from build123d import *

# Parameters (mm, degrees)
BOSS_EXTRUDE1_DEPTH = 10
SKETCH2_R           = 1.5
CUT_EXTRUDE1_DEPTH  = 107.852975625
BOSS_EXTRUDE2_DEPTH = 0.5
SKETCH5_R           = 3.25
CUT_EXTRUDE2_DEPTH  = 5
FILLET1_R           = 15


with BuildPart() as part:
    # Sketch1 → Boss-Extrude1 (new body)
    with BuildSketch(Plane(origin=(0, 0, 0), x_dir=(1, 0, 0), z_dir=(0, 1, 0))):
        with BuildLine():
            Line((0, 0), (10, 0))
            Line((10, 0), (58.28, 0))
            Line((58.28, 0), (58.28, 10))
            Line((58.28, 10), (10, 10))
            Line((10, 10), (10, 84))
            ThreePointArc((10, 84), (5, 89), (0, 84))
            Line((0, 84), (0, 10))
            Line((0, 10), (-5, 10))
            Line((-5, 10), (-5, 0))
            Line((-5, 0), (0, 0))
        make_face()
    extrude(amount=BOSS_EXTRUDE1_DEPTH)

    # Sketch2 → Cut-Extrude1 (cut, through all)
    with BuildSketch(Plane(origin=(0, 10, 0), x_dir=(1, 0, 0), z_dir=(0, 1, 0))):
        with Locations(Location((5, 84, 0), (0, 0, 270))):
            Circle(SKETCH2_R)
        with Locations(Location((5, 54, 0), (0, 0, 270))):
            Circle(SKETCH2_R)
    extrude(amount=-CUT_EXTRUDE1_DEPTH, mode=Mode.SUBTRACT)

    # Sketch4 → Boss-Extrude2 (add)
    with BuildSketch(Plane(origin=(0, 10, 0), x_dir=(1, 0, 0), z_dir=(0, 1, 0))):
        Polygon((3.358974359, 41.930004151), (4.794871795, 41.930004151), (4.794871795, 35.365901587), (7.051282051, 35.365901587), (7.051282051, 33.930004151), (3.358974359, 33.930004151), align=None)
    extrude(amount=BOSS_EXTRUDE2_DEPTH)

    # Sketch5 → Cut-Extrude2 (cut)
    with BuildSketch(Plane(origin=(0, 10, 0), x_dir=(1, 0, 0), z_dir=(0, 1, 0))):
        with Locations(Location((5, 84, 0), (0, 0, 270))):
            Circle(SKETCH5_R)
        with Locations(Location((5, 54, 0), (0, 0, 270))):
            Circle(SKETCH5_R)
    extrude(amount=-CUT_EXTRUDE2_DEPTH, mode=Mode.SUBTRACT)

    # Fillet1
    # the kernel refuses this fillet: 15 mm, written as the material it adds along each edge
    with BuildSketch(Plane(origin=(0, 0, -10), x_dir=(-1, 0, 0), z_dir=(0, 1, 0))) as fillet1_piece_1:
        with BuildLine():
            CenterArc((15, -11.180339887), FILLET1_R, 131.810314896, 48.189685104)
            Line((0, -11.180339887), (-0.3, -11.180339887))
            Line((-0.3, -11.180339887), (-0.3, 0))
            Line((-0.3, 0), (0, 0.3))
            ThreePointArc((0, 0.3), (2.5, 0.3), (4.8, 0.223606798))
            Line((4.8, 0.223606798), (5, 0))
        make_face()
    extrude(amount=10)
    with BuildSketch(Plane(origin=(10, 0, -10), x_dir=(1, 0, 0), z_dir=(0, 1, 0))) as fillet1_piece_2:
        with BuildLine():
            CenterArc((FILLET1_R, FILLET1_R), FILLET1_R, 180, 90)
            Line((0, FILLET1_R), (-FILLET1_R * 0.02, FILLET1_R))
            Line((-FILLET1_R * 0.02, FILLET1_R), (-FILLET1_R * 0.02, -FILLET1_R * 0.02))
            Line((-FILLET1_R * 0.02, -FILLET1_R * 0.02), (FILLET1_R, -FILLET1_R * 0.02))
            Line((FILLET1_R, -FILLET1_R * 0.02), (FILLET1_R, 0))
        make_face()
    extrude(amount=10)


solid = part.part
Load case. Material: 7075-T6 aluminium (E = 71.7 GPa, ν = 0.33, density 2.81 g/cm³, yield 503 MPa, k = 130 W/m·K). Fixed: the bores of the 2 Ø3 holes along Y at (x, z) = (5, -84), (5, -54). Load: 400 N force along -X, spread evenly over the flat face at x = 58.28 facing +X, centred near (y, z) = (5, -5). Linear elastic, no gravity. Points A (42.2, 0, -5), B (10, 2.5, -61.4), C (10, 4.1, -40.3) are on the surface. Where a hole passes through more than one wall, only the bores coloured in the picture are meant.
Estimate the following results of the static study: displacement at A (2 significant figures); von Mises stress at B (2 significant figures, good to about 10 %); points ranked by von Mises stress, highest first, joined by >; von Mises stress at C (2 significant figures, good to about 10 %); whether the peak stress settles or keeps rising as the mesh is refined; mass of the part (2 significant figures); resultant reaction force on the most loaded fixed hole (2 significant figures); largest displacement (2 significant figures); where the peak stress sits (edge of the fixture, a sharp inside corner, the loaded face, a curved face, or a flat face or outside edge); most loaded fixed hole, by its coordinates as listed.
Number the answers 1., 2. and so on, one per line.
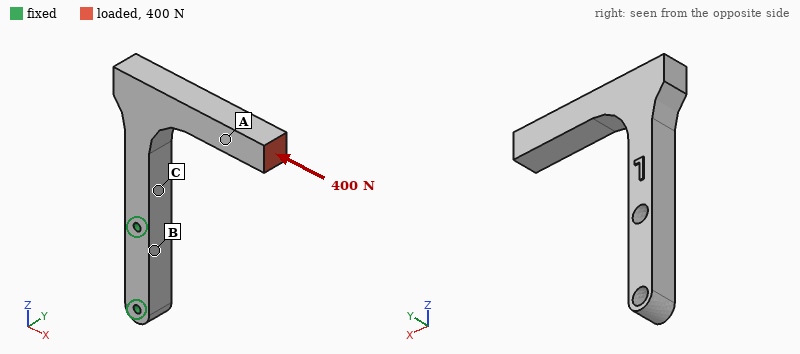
1. 0.52 mm
2. 44 MPa
3. C > B > A
4. 85 MPa
5. keeps rising
6. 40 g
7. 830 N
8. 0.68 mm
9. edge of the fixture
10. (5, -54)
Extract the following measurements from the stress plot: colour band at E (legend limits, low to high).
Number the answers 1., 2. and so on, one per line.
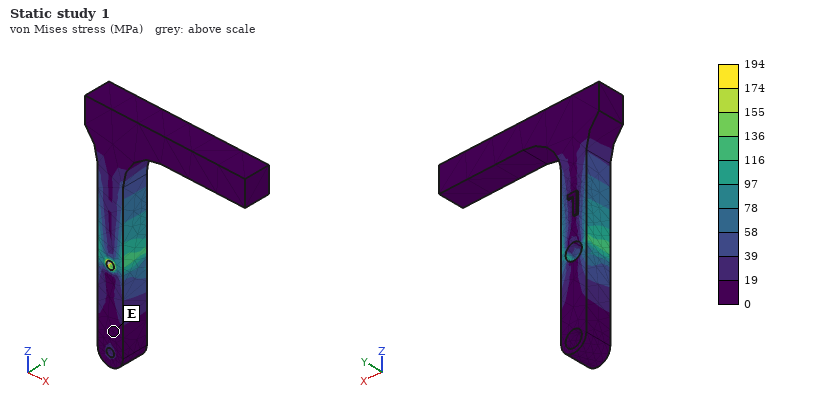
1. 0 to 19 MPa
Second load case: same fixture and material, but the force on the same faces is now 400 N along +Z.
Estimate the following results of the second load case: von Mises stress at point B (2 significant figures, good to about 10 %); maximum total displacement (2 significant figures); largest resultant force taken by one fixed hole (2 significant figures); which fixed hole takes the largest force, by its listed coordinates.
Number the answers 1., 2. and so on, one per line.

1. 48 MPa
2. 1.2 mm
3. 580 N
4. (5, -54)
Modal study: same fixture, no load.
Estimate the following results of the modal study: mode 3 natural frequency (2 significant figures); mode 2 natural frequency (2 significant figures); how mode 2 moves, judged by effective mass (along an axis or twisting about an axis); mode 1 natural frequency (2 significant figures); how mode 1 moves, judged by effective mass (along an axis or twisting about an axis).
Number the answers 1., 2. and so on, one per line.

1. 2000 Hz
2. 910 Hz
3. along X
4. 860 Hz
5. along Y
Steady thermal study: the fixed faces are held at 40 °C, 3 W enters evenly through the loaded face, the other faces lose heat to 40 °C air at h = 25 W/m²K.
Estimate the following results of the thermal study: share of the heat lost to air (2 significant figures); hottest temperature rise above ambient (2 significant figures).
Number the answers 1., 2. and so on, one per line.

1. 29 %
2. 17 K
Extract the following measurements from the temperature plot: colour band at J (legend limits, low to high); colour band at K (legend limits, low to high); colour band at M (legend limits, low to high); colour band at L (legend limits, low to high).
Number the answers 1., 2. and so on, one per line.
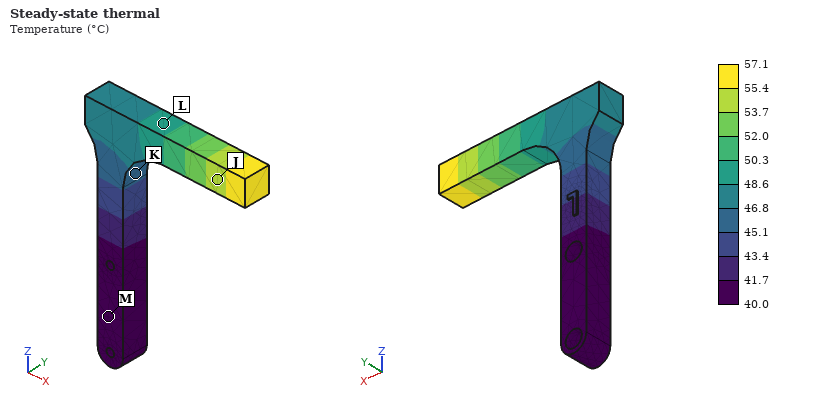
1. 53.7 to 55.4 °C
2. 45.1 to 46.8 °C
3. 40.0 to 41.7 °C
4. 48.6 to 50.3 °C
